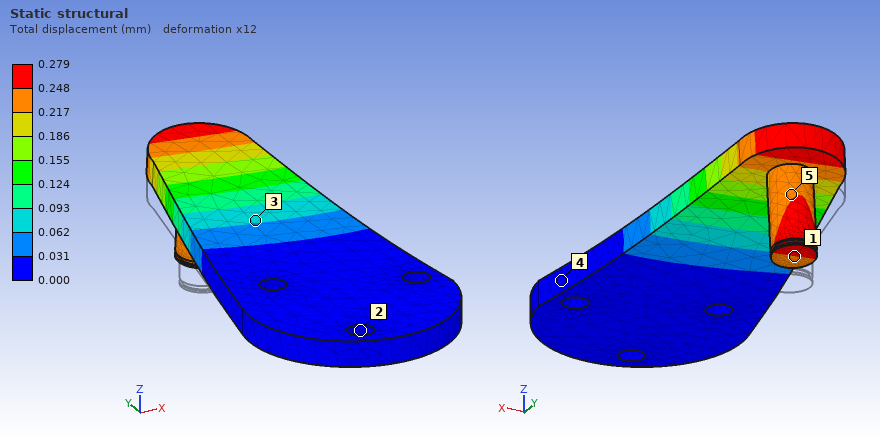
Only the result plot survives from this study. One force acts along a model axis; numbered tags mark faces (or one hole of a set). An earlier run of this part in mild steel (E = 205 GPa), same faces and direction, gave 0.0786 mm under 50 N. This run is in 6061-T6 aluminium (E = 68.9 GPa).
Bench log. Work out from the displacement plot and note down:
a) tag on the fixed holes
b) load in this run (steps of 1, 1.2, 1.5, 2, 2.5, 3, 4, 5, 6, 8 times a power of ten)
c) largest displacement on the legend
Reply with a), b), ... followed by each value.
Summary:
a) 2
b) 60 N
c) 0.279 mm
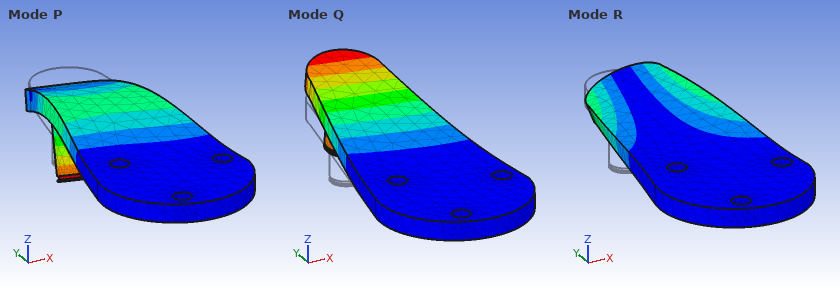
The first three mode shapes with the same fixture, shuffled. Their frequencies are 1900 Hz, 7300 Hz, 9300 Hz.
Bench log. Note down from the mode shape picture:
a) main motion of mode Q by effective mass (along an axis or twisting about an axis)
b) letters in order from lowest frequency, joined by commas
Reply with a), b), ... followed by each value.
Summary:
a) along Z
b) Q, R, P
